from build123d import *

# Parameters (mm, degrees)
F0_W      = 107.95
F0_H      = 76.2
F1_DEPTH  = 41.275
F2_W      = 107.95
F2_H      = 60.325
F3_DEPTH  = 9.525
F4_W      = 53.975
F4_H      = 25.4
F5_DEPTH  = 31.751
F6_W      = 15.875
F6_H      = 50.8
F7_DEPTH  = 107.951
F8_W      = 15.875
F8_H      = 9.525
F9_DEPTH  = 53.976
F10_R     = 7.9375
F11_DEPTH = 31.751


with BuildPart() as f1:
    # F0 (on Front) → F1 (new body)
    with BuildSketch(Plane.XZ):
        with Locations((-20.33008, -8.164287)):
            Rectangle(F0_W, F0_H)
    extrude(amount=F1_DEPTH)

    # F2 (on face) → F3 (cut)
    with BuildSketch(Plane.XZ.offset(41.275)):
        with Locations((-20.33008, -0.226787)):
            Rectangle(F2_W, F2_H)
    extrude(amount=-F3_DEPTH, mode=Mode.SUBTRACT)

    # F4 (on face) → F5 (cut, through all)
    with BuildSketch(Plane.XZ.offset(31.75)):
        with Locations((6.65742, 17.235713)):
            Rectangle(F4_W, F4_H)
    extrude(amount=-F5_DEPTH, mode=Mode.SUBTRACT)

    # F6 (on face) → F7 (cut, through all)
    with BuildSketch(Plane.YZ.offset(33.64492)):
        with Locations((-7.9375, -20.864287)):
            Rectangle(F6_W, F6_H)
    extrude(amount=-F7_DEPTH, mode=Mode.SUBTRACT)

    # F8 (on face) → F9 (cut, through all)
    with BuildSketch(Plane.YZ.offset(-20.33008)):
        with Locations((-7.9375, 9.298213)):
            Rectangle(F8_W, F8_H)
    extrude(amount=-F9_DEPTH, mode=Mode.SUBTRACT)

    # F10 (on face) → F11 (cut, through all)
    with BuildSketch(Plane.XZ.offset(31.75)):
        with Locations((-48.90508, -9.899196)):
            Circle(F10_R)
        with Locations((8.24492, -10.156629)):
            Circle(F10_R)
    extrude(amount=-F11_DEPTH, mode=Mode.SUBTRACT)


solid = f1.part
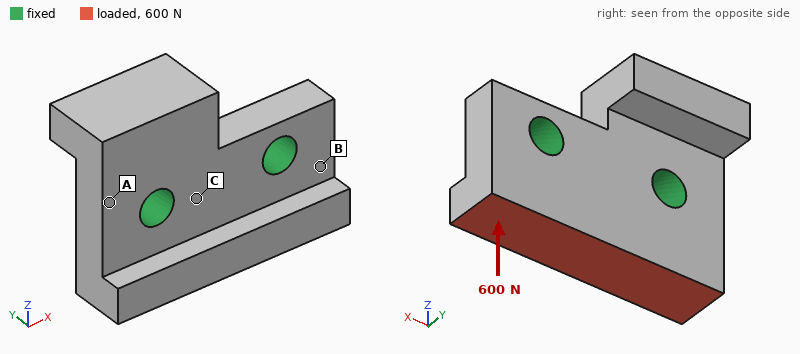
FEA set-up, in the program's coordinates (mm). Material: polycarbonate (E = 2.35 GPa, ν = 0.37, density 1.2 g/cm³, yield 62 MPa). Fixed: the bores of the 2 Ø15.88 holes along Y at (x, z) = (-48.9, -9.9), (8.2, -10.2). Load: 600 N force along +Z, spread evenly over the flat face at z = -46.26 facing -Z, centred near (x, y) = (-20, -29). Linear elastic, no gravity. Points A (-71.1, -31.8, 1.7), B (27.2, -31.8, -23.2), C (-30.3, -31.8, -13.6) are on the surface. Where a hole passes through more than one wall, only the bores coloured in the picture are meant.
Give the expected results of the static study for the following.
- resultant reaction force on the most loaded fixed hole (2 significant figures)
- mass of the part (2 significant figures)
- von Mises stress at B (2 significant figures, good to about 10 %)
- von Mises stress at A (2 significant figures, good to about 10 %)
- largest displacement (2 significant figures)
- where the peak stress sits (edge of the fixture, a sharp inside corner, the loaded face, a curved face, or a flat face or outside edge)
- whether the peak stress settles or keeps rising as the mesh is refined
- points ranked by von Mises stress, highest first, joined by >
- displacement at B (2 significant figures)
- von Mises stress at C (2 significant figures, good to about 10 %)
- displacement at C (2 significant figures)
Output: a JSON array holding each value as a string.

["310 N", "160 g", "0.70 MPa", "0.18 MPa", "27 µm", "edge of the fixture", "keeps rising", "B > C > A", "7.8 µm", "0.45 MPa", "4.1 µm"]
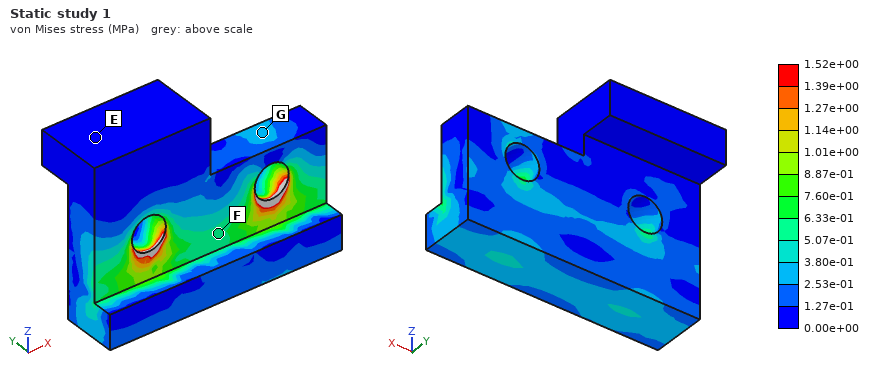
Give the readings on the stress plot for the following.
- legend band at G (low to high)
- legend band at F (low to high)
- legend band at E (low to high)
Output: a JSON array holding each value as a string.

["2.53e-01 to 3.80e-01 MPa", "5.07e-01 to 6.33e-01 MPa", "0.00e+00 to 1.27e-01 MPa"]
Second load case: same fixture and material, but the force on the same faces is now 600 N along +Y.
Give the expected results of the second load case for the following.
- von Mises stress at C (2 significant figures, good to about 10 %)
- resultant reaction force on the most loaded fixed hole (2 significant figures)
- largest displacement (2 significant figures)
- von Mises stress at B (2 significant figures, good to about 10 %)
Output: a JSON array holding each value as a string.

["1.7 MPa", "310 N", "0.13 mm", "2.1 MPa"]
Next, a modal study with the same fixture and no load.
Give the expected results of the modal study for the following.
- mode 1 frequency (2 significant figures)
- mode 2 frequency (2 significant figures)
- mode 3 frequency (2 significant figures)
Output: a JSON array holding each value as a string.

["1500 Hz", "2100 Hz", "2200 Hz"]
